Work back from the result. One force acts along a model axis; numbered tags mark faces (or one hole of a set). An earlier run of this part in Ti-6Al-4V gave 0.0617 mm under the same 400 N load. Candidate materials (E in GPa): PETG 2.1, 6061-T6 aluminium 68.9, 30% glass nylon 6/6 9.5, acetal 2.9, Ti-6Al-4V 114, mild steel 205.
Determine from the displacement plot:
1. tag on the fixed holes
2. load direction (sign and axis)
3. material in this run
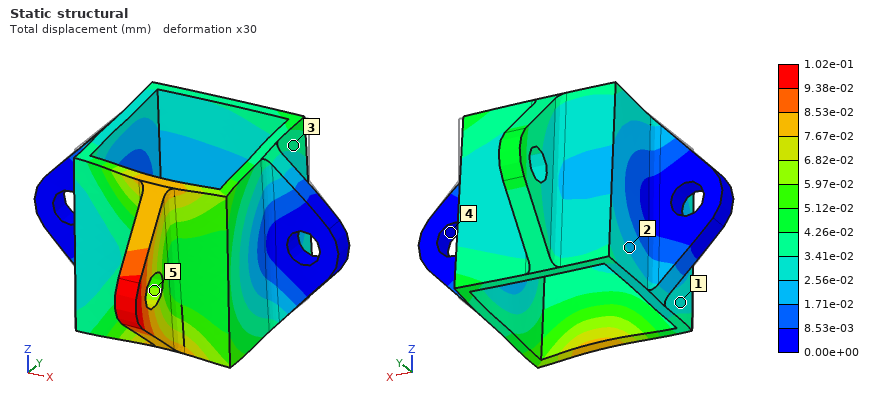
4
-Z
6061-T6 aluminium
